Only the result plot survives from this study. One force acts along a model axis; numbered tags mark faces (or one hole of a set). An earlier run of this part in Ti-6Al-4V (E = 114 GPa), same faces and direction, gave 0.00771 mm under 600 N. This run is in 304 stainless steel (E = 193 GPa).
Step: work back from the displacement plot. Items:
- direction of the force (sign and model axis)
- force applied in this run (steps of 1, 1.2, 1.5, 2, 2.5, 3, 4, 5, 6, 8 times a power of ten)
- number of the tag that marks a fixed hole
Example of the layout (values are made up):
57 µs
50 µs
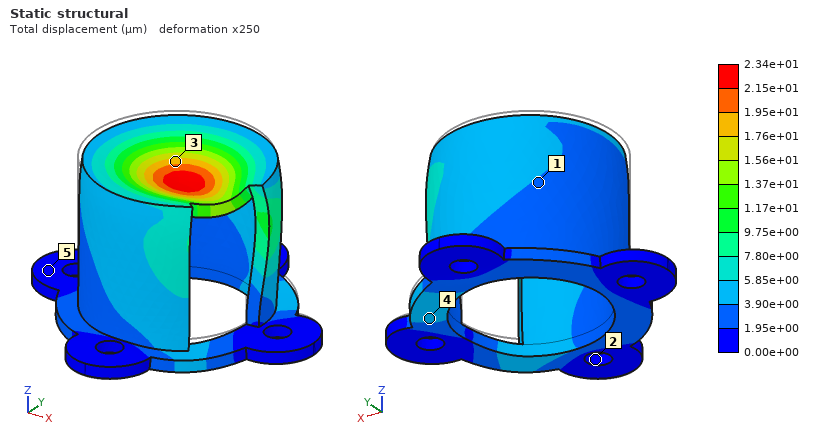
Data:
-Z
3 kN
2
